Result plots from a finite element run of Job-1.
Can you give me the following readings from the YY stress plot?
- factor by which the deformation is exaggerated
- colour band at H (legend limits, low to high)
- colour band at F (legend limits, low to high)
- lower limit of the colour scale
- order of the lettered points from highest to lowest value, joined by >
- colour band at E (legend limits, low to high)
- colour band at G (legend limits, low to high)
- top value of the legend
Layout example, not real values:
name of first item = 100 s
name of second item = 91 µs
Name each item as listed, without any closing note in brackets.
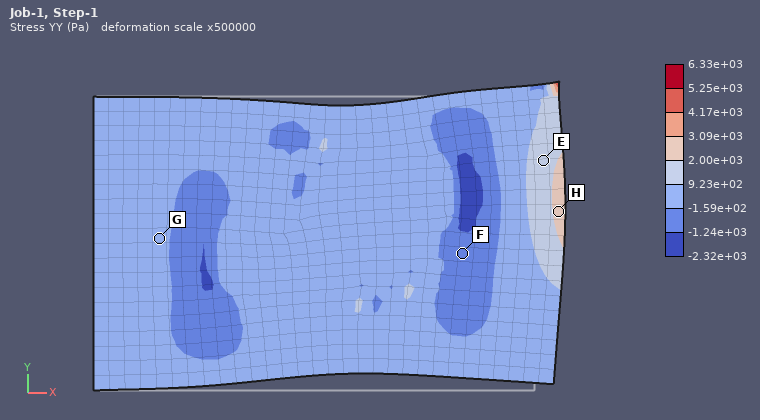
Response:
factor by which the deformation is exaggerated = 500000
colour band at H = 2.00e+03 to 3.09e+03 Pa
colour band at F = -1.24e+03 to -1.59e+02 Pa
lower limit of the colour scale = -2.32e+03 Pa
order of the lettered points from highest to lowest value, joined by > = H > E > G > F
colour band at E = 9.23e+02 to 2.00e+03 Pa
colour band at G = -1.59e+02 to 9.23e+02 Pa
top value of the legend = 6.33e+03 Pa
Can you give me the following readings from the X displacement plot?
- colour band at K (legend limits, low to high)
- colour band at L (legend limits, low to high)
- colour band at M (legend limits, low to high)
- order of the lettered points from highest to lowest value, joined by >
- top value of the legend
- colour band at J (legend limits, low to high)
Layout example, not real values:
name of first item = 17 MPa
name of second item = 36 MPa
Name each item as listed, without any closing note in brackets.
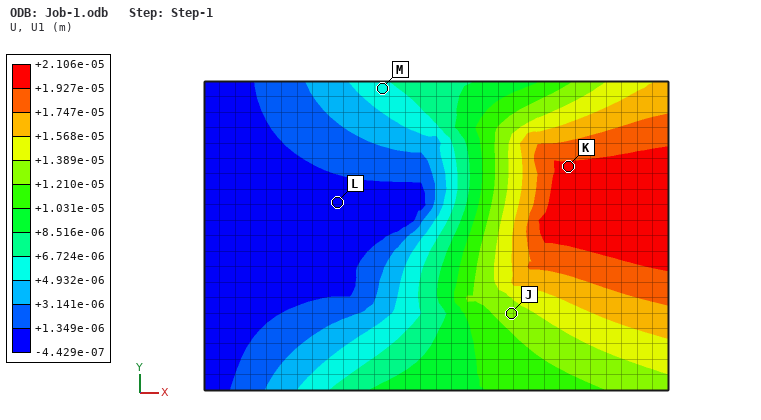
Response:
colour band at K = +1.927e-05 to +2.106e-05 m
colour band at L = -4.429e-07 to +1.349e-06 m
colour band at M = +4.932e-06 to +6.724e-06 m
order of the lettered points from highest to lowest value, joined by > = K > J > M > L
top value of the legend = +2.106e-05 m
colour band at J = +1.210e-05 to +1.389e-05 m
